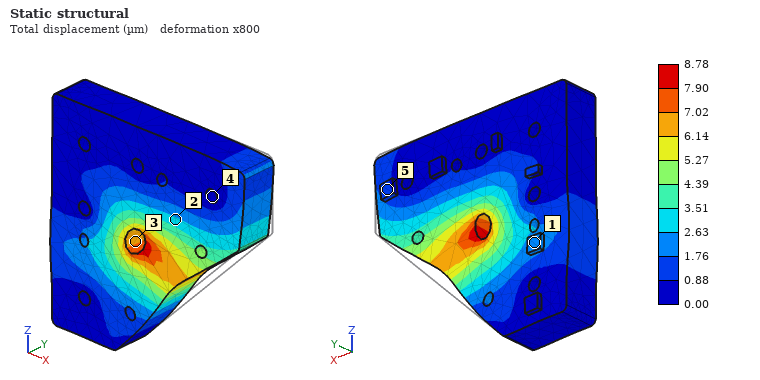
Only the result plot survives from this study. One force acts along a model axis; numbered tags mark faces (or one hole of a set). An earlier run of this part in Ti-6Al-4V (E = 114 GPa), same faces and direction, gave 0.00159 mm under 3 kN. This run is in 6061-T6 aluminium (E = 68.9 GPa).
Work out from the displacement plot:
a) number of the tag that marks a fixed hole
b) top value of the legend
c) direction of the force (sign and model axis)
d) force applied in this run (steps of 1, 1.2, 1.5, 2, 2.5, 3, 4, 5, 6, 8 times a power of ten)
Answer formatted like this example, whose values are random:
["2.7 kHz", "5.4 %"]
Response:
["4", "8.78 µm", "-X", "10 kN"]
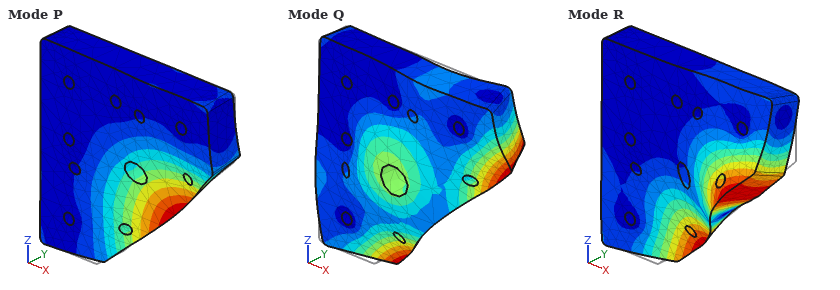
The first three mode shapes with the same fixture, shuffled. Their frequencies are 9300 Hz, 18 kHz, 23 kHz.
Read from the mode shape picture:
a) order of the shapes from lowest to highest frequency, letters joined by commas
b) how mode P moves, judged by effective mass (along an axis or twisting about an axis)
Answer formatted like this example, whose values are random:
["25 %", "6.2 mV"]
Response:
["P, R, Q", "along Y"]
